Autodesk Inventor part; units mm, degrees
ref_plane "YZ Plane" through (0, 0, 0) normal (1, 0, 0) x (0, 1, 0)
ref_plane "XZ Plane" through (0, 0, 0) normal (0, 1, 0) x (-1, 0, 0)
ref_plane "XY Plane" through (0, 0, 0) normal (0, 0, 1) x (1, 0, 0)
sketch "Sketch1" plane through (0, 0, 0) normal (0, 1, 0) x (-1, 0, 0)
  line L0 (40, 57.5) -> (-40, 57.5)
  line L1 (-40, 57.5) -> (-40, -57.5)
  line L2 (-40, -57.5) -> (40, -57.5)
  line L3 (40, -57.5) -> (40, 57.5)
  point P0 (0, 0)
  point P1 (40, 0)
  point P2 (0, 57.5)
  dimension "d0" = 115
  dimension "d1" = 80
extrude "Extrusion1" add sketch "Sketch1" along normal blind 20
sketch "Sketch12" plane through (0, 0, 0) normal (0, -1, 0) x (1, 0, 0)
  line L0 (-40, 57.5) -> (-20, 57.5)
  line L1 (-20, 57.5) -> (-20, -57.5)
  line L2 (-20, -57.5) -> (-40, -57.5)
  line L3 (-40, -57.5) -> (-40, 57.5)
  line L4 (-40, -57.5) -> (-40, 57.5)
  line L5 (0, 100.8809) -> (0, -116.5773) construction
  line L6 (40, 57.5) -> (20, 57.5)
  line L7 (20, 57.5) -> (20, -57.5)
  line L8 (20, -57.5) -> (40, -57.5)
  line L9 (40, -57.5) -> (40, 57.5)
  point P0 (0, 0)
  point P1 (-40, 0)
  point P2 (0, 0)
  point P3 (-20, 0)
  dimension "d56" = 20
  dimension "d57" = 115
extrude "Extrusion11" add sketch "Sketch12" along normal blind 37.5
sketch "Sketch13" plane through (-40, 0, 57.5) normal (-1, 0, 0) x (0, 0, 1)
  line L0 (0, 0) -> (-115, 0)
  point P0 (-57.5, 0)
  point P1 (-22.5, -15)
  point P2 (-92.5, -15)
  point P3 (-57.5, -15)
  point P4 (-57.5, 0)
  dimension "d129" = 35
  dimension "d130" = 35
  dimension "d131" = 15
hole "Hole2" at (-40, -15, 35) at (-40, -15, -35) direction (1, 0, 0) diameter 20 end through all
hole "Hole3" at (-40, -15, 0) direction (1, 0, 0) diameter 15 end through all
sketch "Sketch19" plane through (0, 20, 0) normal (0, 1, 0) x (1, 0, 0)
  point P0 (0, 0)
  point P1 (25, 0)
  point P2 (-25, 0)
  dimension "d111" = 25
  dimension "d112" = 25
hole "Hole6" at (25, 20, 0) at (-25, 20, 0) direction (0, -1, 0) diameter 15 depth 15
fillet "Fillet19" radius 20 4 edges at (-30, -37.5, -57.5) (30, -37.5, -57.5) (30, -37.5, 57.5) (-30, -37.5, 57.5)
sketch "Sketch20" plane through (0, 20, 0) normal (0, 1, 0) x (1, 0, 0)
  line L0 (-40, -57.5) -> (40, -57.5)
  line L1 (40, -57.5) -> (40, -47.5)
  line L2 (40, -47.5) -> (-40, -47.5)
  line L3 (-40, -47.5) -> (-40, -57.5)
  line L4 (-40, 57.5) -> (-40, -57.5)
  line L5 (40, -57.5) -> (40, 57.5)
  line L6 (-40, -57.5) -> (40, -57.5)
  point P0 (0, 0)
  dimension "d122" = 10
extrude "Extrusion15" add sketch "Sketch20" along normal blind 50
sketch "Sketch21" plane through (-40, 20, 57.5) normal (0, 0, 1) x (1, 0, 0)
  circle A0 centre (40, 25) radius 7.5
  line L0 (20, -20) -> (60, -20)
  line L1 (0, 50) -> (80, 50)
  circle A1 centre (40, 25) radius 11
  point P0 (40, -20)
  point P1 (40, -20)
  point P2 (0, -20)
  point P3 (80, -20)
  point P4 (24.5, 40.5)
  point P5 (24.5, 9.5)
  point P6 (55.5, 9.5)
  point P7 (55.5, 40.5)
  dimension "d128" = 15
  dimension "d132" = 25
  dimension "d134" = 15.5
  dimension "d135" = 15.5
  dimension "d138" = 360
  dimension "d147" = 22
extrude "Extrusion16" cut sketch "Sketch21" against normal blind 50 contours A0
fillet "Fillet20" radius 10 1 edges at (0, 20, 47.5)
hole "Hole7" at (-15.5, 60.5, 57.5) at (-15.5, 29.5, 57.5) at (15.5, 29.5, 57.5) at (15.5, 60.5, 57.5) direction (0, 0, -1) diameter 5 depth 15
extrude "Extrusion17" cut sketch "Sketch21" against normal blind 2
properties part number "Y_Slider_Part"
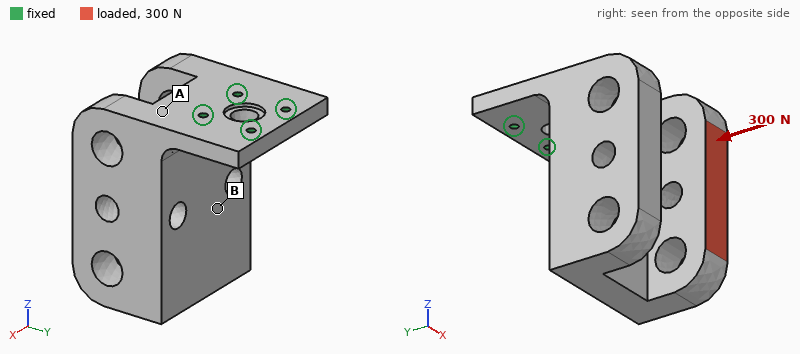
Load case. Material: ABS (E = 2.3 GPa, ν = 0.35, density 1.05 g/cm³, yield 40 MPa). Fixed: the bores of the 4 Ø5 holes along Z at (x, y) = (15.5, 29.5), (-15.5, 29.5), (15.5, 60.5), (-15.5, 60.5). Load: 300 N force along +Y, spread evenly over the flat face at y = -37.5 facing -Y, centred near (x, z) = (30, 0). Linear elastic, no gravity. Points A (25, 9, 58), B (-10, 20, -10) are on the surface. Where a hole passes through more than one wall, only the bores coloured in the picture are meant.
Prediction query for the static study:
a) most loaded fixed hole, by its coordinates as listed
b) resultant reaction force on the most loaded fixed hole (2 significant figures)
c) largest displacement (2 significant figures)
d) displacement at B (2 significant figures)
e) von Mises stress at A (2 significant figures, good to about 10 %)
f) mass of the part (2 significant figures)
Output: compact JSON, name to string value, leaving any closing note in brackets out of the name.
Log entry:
{"most loaded fixed hole, by its coordinates as listed": "(15.5, 29.5)", "resultant reaction force on the most loaded fixed hole": "300 N", "largest displacement": "1.6 mm", "displacement at B": "0.76 mm", "von Mises stress at A": "1.9 MPa", "mass of the part": "370 g"}
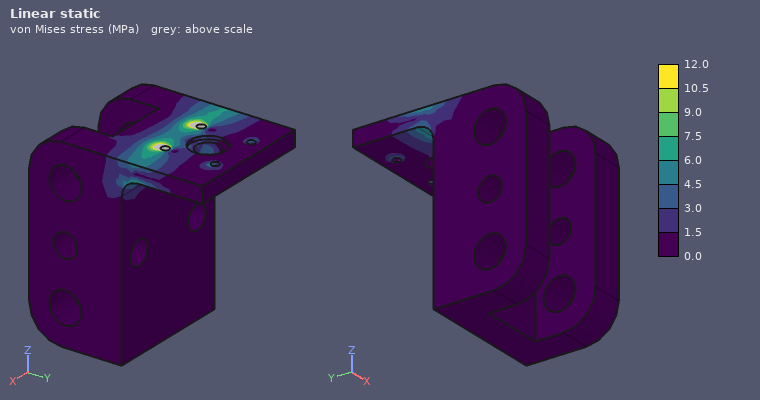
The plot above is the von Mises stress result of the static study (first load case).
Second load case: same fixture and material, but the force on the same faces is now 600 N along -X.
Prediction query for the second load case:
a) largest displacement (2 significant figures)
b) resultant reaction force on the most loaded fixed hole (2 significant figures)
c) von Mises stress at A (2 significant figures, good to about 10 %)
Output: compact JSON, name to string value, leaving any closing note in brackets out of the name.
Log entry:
{"largest displacement": "0.89 mm", "resultant reaction force on the most loaded fixed hole": "1.2 kN", "von Mises stress at A": "2.5 MPa"}
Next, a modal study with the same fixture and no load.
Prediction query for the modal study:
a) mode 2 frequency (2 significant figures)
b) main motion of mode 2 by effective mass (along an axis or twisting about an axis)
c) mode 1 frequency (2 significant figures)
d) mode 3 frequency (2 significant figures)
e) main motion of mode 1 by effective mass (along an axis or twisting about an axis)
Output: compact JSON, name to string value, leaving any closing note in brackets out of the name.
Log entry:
{"mode 2 frequency": "320 Hz", "main motion of mode 2 by effective mass": "along X", "mode 1 frequency": "140 Hz", "mode 3 frequency": "590 Hz", "main motion of mode 1 by effective mass": "along Y"}
